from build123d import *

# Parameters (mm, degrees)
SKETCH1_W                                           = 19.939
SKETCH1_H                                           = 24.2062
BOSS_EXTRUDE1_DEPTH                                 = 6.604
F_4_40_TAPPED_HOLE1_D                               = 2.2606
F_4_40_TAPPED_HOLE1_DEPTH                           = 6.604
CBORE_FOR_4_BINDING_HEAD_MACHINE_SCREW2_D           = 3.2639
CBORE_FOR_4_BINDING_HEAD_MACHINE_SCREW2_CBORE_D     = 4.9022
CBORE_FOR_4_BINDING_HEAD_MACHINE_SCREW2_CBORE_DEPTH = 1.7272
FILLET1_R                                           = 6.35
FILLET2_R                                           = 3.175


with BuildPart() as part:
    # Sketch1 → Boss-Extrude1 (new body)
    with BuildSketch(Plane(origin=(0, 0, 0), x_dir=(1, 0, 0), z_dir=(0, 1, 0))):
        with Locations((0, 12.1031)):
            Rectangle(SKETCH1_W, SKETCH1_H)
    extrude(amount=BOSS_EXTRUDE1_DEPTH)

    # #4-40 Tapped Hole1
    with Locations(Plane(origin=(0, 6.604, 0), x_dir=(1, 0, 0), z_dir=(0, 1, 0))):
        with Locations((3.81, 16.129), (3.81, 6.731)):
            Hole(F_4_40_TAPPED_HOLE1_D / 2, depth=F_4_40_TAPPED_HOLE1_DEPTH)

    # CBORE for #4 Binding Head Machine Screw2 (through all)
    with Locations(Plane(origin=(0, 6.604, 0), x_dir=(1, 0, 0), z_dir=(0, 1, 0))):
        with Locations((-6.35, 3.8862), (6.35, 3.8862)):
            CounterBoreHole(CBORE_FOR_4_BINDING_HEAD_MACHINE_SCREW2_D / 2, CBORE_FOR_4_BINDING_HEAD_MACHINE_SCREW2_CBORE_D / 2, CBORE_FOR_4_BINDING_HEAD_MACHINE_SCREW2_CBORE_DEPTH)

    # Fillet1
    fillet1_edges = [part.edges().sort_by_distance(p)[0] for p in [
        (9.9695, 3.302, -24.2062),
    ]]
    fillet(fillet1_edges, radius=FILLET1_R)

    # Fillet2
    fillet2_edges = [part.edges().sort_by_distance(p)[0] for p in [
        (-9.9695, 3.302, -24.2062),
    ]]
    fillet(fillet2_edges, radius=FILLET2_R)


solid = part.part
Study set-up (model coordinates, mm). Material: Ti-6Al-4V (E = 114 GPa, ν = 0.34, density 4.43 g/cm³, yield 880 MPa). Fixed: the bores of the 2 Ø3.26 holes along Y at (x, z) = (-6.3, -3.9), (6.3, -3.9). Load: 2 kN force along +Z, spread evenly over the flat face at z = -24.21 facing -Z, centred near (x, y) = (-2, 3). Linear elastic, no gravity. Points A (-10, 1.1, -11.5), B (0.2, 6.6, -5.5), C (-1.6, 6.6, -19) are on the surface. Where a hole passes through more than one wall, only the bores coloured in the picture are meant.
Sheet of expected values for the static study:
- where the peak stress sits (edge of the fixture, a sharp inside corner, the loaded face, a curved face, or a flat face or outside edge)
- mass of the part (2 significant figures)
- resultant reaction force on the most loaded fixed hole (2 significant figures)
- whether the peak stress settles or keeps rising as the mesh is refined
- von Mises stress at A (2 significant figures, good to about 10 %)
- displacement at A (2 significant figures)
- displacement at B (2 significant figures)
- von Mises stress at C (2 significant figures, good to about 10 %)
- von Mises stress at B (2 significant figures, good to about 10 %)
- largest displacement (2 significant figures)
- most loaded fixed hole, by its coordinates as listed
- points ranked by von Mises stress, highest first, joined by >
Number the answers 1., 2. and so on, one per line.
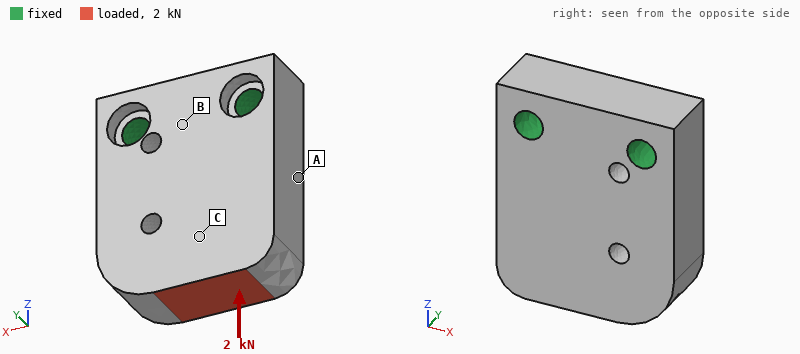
1. edge of the fixture
2. 13 g
3. 1.3 kN
4. keeps rising
5. 20 MPa
6. 1.9 µm
7. 1.5 µm
8. 28 MPa
9. 7.4 MPa
10. 6.2 µm
11. (-6.3, -3.9)
12. C > A > B
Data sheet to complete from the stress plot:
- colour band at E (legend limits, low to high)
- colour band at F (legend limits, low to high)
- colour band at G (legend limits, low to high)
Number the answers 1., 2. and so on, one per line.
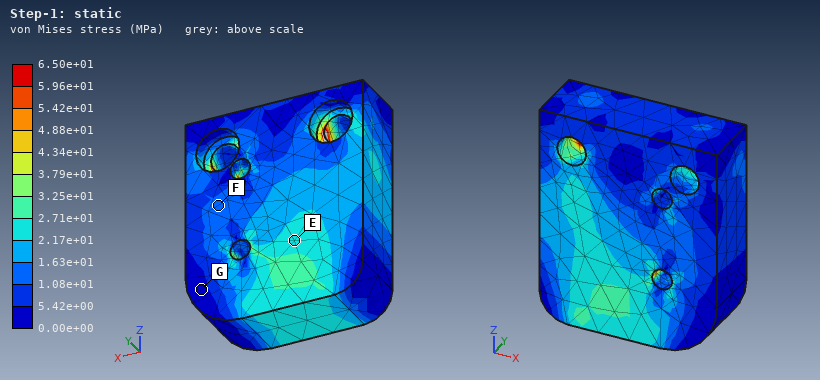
1. 2.17e+01 to 2.71e+01 MPa
2. 1.08e+01 to 1.63e+01 MPa
3. 0.00e+00 to 5.42e+00 MPa
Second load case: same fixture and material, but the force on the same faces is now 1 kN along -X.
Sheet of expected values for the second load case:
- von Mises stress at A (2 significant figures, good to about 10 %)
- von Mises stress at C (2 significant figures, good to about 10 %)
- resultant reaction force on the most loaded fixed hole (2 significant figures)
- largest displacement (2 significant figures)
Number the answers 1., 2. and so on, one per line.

1. 30 MPa
2. 17 MPa
3. 1.5 kN
4. 12 µm
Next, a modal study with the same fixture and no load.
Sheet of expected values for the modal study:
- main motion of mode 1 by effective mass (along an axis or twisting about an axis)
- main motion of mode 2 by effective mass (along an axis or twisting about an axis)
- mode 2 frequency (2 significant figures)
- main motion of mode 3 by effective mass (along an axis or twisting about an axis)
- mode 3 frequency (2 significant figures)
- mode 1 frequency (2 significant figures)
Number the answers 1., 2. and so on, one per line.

1. along Y
2. along X
3. 24 kHz
4. along X
5. 26 kHz
6. 11 kHz
